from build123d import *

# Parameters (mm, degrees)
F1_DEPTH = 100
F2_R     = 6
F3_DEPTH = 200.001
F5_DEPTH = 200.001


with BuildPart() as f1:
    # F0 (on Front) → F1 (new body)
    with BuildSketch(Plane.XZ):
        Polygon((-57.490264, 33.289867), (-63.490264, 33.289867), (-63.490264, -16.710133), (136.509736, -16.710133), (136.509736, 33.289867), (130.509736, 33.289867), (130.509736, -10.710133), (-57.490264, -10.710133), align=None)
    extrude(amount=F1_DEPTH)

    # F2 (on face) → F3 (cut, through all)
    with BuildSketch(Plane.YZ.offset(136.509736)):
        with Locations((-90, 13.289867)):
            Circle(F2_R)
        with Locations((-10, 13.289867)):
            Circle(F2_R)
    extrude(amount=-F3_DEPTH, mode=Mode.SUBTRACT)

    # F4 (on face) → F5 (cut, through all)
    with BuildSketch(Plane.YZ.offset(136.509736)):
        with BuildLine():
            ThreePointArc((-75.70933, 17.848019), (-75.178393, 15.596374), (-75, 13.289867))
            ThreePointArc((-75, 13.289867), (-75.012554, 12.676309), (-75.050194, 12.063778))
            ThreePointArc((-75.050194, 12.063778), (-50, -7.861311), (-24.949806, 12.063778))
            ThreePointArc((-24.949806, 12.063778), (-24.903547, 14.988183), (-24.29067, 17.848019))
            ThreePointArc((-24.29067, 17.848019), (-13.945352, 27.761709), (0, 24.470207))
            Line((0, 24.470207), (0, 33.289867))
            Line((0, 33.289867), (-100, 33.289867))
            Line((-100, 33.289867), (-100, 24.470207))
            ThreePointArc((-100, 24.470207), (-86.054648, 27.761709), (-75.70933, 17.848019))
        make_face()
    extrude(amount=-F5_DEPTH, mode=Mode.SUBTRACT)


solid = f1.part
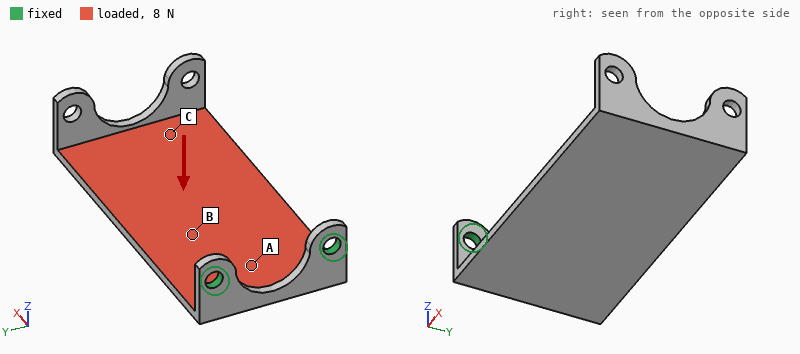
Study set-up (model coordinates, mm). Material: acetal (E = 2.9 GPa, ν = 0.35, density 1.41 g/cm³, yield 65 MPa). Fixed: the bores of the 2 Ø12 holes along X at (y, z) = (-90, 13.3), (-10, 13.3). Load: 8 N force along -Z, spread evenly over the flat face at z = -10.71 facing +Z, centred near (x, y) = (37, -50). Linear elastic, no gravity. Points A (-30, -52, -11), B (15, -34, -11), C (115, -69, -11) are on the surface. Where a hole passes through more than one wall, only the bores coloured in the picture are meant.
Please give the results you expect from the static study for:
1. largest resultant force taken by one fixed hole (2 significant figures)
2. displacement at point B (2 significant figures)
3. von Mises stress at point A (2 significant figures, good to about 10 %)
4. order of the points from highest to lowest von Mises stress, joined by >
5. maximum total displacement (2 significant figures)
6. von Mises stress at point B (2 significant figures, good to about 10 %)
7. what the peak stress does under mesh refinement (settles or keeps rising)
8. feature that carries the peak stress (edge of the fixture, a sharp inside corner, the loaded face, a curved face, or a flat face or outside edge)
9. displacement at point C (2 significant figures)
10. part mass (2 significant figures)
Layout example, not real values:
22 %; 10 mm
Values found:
4.7 N; 0.69 mm; 0.83 MPa; A > B > C; 2.4 mm; 0.46 MPa; keeps rising; edge of the fixture; 2.0 mm; 200 g
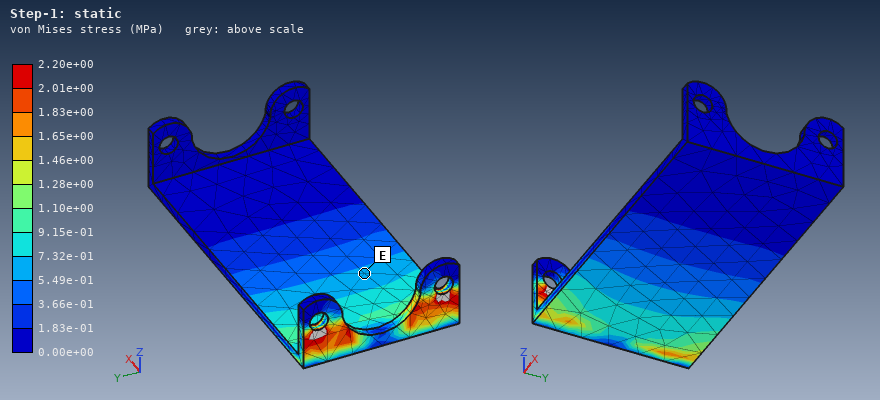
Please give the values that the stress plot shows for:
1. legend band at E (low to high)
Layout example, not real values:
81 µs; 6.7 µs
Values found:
5.49e-01 to 7.32e-01 MPa
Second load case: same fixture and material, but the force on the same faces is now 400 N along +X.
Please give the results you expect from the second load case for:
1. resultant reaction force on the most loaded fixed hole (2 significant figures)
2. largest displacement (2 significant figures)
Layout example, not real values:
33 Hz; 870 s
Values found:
200 N; 2.2 mm
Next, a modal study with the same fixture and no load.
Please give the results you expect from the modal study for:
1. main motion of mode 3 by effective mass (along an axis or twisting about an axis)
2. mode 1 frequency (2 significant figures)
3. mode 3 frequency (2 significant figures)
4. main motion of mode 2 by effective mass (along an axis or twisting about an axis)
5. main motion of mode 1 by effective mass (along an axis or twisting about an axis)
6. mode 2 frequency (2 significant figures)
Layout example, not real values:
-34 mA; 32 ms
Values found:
along Y; 24 Hz; 150 Hz; along Y; along Z; 100 Hz
